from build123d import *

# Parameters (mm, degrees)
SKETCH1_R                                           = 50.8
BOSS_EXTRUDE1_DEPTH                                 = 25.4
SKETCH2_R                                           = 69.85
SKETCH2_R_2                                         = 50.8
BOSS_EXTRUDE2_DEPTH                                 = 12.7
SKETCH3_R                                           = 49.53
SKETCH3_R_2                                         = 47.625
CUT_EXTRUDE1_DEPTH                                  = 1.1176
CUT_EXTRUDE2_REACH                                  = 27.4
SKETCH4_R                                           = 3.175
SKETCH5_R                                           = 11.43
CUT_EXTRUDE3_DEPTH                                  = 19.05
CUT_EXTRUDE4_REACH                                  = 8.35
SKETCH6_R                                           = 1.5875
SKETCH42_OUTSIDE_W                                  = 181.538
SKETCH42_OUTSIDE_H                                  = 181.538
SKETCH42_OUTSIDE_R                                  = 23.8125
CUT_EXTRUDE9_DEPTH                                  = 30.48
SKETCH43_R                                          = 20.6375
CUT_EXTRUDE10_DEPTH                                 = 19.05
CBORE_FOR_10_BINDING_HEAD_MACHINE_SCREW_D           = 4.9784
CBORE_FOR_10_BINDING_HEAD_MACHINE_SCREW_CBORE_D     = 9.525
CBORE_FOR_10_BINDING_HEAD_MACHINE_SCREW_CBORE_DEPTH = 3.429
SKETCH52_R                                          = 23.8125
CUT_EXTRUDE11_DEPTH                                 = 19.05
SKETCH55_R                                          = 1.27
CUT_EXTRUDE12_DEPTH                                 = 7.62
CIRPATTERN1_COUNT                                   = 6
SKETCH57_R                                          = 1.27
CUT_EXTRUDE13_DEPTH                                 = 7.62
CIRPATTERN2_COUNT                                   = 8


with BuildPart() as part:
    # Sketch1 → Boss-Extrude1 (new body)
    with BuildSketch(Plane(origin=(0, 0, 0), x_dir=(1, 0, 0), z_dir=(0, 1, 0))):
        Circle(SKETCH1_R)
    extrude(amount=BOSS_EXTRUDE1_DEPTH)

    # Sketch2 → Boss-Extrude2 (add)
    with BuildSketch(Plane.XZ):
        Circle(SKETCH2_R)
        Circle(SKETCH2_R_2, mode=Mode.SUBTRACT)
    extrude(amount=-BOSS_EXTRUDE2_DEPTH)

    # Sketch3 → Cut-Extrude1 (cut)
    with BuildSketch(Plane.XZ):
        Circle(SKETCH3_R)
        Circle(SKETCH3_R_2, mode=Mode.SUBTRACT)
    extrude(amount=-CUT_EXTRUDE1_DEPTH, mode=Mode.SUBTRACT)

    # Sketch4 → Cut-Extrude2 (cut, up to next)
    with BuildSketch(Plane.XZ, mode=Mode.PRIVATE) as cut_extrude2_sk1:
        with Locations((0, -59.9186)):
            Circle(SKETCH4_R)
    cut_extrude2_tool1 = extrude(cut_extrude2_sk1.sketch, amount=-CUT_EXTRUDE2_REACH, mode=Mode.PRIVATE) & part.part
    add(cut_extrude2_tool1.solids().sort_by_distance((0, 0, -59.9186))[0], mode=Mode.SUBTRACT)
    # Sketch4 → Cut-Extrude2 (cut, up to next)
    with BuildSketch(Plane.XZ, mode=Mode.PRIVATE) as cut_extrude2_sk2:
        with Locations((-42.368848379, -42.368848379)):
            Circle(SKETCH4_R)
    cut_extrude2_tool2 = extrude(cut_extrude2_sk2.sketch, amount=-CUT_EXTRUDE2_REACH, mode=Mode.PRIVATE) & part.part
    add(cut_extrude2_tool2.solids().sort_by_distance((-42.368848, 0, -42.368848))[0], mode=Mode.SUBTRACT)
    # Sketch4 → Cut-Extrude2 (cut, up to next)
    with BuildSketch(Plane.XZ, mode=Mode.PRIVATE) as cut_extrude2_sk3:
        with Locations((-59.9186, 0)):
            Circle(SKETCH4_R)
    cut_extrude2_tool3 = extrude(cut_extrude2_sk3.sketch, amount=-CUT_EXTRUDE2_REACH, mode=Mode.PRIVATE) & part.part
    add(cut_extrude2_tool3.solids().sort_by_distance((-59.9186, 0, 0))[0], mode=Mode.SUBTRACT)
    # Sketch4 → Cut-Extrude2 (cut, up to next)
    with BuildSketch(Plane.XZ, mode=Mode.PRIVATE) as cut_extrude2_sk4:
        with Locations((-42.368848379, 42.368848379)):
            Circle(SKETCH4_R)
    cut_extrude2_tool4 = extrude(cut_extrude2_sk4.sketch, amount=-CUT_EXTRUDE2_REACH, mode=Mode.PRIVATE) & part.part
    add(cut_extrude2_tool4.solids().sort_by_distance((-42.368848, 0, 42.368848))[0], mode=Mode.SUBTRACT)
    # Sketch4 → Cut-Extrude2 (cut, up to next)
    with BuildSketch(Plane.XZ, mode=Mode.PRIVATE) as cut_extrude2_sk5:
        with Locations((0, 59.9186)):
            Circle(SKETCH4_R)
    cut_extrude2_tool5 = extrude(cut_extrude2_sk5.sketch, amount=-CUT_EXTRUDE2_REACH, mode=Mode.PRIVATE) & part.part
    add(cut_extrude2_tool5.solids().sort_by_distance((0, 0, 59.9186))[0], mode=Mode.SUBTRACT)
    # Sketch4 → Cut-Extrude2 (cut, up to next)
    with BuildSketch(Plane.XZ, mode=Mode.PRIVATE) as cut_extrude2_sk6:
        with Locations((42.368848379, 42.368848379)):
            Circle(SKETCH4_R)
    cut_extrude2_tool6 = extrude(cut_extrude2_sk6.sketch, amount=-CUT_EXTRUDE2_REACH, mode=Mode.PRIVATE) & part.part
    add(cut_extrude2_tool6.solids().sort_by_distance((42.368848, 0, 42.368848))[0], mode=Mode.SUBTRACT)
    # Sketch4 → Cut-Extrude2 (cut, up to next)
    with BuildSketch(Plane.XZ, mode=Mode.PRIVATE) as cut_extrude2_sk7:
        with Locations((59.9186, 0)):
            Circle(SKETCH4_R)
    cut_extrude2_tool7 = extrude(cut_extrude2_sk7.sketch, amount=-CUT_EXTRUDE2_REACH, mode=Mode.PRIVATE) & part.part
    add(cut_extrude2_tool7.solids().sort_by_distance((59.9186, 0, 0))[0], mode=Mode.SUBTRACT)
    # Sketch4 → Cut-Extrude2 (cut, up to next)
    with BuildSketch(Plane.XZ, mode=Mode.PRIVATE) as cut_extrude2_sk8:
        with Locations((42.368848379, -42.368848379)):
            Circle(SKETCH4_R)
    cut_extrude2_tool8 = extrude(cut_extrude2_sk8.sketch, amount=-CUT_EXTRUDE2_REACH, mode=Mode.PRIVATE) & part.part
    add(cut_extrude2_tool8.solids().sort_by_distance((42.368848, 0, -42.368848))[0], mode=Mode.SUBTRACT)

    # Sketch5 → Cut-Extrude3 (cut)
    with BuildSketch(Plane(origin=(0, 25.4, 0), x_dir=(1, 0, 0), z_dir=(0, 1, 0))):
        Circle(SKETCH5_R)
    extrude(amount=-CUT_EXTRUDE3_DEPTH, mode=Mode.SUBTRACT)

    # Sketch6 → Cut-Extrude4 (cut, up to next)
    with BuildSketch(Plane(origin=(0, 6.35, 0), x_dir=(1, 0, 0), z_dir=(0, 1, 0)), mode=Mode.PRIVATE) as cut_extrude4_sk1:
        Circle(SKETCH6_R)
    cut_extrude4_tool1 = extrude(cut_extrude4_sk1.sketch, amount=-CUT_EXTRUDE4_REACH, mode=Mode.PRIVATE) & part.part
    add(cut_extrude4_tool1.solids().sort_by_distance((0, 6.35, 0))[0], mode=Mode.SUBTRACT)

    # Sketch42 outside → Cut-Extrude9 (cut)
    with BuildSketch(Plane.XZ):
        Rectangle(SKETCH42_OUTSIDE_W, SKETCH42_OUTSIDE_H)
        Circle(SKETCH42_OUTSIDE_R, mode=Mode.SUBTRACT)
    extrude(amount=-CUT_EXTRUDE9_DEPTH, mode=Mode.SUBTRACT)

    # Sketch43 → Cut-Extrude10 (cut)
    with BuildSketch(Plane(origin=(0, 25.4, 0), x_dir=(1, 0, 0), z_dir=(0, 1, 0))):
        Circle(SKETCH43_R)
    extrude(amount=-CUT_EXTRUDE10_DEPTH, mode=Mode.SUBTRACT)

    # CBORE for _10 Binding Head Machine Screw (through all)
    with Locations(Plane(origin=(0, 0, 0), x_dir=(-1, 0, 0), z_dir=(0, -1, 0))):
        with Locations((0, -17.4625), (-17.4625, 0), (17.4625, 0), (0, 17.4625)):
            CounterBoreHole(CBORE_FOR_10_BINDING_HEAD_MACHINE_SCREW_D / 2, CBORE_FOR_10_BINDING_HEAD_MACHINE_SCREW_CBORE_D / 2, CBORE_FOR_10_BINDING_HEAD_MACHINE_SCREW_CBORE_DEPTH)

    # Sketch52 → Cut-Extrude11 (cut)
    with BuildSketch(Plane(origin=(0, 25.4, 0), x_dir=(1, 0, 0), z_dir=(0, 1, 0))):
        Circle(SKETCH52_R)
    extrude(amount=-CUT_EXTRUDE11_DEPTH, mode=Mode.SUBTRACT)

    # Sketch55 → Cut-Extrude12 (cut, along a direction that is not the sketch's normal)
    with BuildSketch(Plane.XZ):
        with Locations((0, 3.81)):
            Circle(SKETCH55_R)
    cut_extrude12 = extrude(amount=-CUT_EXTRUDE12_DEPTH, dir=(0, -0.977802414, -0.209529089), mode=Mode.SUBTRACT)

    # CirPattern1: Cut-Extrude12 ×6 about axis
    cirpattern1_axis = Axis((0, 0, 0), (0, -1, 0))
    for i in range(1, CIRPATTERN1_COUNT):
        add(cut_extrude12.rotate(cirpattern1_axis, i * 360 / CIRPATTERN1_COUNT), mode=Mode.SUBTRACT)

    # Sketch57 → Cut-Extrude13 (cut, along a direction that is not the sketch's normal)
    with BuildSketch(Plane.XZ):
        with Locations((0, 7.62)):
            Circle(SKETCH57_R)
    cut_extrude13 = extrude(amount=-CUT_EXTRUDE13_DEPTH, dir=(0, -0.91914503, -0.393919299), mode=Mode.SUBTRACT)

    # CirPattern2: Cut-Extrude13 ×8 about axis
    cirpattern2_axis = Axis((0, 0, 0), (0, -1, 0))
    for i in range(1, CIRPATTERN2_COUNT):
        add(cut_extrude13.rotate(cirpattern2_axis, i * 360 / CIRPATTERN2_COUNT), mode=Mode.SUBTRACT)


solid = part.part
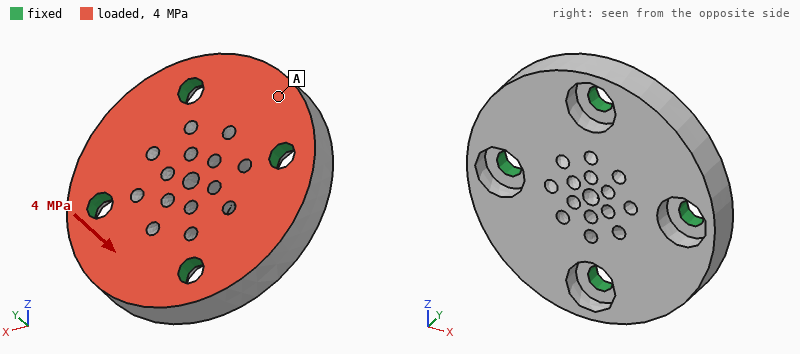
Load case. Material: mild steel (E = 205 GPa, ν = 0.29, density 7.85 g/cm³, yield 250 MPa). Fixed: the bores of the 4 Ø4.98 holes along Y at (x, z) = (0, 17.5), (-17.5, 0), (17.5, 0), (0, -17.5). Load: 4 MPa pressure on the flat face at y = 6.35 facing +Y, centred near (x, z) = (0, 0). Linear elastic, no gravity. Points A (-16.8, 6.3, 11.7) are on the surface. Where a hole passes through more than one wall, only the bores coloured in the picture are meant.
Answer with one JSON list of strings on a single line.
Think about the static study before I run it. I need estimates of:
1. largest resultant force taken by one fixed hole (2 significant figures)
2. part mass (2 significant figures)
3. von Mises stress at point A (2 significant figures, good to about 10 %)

["1.6 kN", "75 g", "14 MPa"]
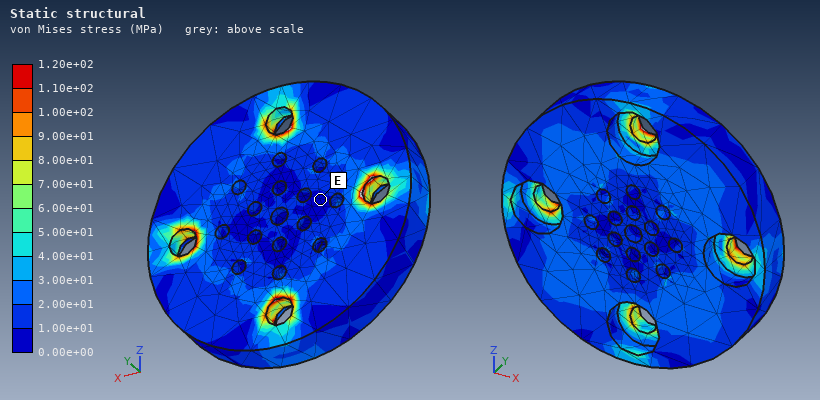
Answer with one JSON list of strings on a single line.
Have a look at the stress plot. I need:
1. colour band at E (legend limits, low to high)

["0.00e+00 to 1.00e+01 MPa"]
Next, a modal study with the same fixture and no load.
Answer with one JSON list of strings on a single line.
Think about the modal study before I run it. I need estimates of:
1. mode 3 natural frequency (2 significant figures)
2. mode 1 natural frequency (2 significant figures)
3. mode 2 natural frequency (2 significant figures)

["23 kHz", "21 kHz", "23 kHz"]
